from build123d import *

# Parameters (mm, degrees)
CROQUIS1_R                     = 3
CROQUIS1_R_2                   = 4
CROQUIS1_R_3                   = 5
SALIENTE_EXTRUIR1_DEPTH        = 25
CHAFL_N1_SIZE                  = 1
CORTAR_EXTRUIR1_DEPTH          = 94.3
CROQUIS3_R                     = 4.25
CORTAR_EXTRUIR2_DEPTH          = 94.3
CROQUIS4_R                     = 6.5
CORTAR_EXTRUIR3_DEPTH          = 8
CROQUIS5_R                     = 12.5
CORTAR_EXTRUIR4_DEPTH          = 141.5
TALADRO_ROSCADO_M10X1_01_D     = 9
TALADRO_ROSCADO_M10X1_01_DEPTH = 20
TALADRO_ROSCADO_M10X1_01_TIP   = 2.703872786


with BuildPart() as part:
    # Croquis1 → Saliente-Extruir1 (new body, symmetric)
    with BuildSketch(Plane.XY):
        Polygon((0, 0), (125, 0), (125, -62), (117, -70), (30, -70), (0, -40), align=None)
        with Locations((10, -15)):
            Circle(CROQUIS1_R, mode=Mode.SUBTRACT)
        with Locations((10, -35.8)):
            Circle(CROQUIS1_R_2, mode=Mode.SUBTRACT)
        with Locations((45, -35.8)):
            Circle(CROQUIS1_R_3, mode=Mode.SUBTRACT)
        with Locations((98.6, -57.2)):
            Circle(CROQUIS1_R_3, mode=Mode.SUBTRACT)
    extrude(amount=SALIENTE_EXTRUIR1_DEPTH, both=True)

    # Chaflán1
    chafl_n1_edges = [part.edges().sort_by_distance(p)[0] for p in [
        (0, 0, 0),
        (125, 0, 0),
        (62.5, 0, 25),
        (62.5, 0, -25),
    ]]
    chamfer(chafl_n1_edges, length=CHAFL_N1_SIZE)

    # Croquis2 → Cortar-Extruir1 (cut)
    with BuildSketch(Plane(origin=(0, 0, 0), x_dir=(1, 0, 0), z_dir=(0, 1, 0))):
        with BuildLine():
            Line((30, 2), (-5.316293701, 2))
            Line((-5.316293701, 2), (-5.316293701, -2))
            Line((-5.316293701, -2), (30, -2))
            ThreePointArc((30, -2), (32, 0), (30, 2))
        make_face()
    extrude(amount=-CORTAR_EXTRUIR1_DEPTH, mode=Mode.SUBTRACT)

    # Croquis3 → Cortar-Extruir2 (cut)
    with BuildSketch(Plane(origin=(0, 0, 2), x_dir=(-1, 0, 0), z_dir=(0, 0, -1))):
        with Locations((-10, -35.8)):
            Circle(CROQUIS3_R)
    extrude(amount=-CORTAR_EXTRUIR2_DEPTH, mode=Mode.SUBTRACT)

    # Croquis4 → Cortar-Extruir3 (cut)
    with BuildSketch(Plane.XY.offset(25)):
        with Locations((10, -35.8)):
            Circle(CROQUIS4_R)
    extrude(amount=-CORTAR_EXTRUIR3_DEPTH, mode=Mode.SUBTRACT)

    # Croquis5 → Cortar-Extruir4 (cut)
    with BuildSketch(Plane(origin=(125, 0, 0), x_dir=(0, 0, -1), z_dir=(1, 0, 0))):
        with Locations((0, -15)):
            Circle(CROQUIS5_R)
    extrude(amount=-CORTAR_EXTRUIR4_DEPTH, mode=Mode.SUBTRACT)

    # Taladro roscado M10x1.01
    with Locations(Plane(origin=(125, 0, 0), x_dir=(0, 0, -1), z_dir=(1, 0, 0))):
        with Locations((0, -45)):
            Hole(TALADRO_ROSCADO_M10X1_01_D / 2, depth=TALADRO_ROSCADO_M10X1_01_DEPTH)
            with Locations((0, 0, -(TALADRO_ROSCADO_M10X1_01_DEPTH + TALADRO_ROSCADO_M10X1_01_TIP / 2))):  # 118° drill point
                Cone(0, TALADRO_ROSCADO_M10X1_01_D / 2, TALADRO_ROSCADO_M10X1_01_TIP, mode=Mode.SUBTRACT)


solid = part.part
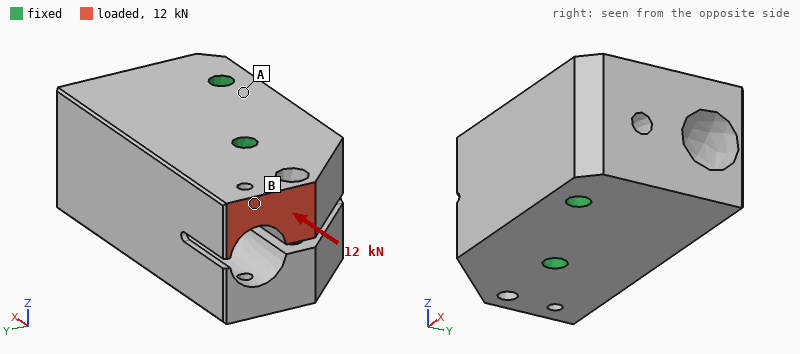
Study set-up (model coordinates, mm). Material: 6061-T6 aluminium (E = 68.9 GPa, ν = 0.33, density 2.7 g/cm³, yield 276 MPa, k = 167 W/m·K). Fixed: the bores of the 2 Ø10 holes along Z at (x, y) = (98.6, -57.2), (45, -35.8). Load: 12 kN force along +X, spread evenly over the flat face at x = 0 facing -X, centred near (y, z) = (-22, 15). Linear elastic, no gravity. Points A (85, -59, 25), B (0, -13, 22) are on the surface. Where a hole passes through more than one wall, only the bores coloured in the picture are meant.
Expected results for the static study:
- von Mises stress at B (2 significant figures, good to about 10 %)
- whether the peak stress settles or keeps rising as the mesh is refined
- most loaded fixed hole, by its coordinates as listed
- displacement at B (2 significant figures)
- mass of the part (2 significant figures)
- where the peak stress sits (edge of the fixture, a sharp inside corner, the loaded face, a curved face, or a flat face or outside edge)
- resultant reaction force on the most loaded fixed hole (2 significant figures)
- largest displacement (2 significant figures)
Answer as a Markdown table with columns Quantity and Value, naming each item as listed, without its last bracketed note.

| Quantity | Value |
|---|---|
| von Mises stress at B | 14 MPa |
| whether the peak stress settles or keeps rising as the mesh is refined | keeps rising |
| most loaded fixed hole, by its coordinates as listed | (45, -35.8) |
| displacement at B | 24 µm |
| mass of the part | 900 g |
| where the peak stress sits | a sharp inside corner |
| resultant reaction force on the most loaded fixed hole | 11 kN |
| largest displacement | 25 µm |
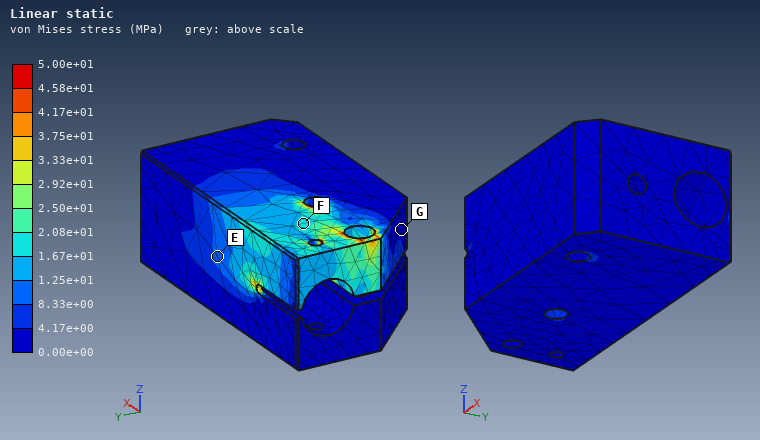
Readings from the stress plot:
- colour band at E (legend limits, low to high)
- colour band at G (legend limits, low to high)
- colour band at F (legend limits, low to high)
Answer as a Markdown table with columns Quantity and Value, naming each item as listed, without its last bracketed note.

| Quantity | Value |
|---|---|
| colour band at E | 8.33e+00 to 1.25e+01 MPa |
| colour band at G | 0.00e+00 to 4.17e+00 MPa |
| colour band at F | 1.67e+01 to 2.08e+01 MPa |
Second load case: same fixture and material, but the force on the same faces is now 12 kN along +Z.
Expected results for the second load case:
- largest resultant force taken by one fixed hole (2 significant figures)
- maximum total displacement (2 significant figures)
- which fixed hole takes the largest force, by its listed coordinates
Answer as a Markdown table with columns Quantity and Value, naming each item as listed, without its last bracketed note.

| Quantity | Value |
|---|---|
| largest resultant force taken by one fixed hole | 14 kN |
| maximum total displacement | 0.20 mm |
| which fixed hole takes the largest force, by its listed coordinates | (45, -35.8) |
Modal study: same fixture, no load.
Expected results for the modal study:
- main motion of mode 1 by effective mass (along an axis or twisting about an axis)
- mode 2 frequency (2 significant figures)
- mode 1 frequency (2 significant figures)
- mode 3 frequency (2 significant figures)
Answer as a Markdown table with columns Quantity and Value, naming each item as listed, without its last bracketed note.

| Quantity | Value |
|---|---|
| main motion of mode 1 by effective mass | along Z |
| mode 2 frequency | 8900 Hz |
| mode 1 frequency | 8100 Hz |
| mode 3 frequency | 9200 Hz |
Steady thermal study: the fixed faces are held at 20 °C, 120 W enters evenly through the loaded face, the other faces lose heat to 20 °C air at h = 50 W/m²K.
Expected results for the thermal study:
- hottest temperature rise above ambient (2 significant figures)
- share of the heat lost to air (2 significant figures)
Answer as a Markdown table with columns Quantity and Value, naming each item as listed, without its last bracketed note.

| Quantity | Value |
|---|---|
| hottest temperature rise above ambient | 41 K |
| share of the heat lost to air | 7.5 % |
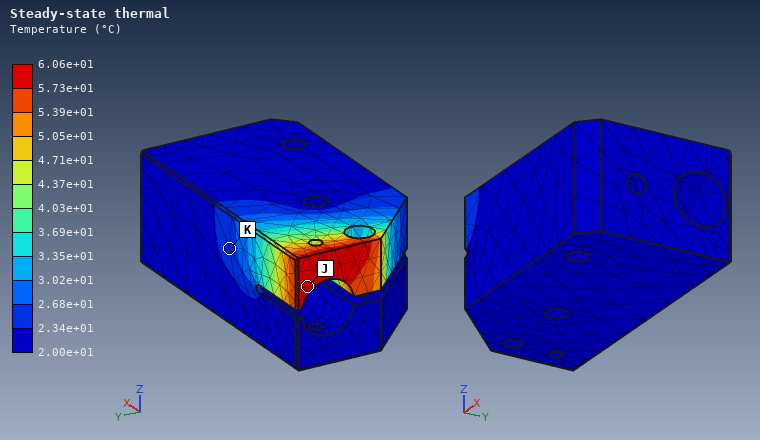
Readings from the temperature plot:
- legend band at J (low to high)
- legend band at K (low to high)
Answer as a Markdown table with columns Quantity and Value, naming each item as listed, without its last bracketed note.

| Quantity | Value |
|---|---|
| legend band at J | 5.73e+01 to 6.06e+01 °C |
| legend band at K | 2.34e+01 to 2.68e+01 °C |
